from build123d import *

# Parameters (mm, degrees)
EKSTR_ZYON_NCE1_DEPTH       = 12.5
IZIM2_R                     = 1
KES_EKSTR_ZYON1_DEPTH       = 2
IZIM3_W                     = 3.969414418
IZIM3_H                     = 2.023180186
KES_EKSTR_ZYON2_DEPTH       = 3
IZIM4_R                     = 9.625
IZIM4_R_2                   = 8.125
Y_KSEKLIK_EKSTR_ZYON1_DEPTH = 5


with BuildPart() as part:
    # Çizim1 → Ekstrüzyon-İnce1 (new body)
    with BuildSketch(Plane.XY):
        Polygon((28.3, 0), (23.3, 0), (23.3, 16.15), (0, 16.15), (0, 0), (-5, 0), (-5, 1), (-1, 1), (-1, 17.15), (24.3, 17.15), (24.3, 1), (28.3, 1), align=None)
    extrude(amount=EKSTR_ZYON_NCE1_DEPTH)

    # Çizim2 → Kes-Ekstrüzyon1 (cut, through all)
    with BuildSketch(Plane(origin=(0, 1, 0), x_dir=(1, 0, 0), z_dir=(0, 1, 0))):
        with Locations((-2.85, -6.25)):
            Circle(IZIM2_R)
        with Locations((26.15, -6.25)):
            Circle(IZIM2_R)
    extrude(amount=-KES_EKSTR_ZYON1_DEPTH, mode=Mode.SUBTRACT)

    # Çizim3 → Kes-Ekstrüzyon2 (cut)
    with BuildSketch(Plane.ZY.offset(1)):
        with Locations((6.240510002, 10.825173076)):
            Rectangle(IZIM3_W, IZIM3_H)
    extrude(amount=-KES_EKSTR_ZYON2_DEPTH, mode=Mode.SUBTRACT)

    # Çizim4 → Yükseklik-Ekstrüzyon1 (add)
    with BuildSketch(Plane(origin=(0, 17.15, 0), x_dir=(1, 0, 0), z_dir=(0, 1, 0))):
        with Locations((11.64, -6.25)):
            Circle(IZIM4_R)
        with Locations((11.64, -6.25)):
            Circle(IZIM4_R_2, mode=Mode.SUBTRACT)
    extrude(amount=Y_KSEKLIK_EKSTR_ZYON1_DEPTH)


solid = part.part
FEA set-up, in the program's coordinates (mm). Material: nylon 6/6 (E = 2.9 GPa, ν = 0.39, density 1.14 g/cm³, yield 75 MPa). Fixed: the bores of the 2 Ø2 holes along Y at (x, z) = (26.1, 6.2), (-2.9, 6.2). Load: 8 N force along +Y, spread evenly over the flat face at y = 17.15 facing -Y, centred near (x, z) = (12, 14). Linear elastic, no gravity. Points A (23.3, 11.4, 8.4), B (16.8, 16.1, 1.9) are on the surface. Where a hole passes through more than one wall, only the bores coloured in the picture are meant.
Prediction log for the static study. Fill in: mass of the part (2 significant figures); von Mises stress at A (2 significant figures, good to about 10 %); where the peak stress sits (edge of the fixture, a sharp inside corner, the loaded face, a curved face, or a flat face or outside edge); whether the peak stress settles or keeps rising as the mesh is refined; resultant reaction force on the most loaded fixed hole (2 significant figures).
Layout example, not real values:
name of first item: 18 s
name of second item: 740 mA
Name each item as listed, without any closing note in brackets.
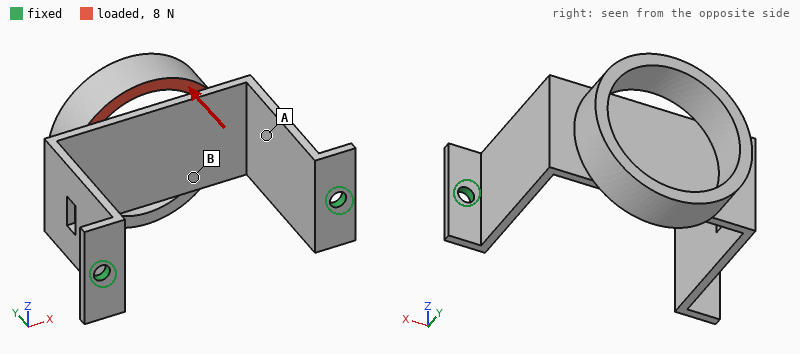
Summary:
mass of the part: 1.4 g
von Mises stress at A: 2.7 MPa
where the peak stress sits: edge of the fixture
whether the peak stress settles or keeps rising as the mesh is refined: keeps rising
resultant reaction force on the most loaded fixed hole: 4.1 N
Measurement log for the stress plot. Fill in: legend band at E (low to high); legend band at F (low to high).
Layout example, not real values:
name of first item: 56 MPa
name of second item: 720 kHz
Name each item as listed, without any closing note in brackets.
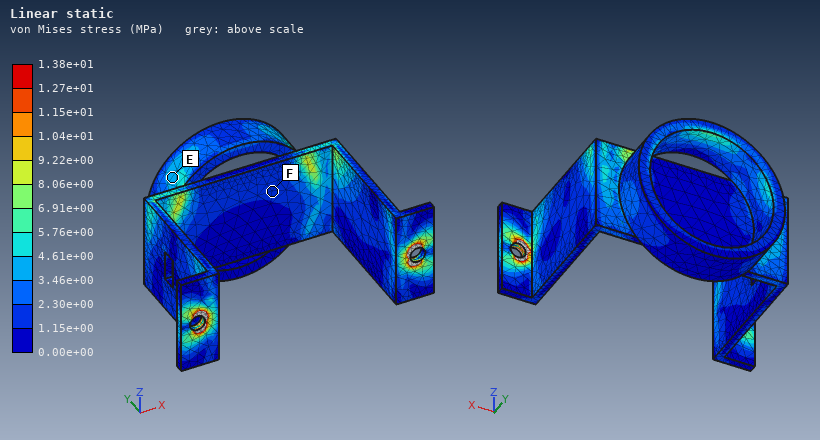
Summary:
legend band at E: 3.46e+00 to 4.61e+00 MPa
legend band at F: 1.15e+00 to 2.30e+00 MPa
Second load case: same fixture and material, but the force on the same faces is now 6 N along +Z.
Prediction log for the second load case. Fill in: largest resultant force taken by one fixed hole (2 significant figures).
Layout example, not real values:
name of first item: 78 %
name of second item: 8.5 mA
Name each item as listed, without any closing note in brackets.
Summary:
largest resultant force taken by one fixed hole: 3.0 N
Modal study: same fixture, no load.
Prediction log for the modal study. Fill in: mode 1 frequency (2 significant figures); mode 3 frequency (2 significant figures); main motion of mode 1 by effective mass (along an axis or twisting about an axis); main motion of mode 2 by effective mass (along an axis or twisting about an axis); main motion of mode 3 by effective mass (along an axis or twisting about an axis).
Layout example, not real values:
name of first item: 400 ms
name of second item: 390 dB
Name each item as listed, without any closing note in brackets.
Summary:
mode 1 frequency: 530 Hz
mode 3 frequency: 1300 Hz
main motion of mode 1 by effective mass: along X
main motion of mode 2 by effective mass: along Z
main motion of mode 3 by effective mass: twisting about Y
